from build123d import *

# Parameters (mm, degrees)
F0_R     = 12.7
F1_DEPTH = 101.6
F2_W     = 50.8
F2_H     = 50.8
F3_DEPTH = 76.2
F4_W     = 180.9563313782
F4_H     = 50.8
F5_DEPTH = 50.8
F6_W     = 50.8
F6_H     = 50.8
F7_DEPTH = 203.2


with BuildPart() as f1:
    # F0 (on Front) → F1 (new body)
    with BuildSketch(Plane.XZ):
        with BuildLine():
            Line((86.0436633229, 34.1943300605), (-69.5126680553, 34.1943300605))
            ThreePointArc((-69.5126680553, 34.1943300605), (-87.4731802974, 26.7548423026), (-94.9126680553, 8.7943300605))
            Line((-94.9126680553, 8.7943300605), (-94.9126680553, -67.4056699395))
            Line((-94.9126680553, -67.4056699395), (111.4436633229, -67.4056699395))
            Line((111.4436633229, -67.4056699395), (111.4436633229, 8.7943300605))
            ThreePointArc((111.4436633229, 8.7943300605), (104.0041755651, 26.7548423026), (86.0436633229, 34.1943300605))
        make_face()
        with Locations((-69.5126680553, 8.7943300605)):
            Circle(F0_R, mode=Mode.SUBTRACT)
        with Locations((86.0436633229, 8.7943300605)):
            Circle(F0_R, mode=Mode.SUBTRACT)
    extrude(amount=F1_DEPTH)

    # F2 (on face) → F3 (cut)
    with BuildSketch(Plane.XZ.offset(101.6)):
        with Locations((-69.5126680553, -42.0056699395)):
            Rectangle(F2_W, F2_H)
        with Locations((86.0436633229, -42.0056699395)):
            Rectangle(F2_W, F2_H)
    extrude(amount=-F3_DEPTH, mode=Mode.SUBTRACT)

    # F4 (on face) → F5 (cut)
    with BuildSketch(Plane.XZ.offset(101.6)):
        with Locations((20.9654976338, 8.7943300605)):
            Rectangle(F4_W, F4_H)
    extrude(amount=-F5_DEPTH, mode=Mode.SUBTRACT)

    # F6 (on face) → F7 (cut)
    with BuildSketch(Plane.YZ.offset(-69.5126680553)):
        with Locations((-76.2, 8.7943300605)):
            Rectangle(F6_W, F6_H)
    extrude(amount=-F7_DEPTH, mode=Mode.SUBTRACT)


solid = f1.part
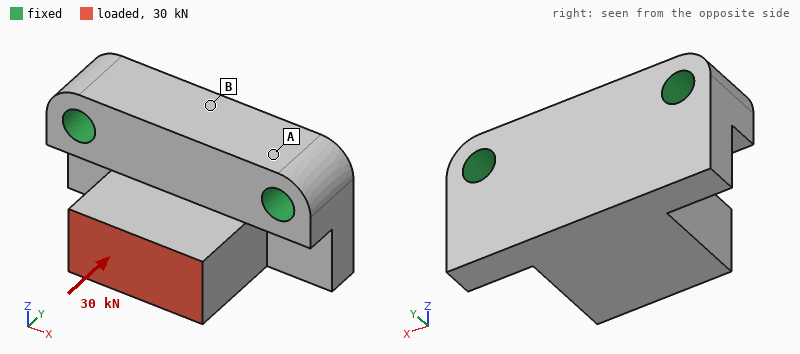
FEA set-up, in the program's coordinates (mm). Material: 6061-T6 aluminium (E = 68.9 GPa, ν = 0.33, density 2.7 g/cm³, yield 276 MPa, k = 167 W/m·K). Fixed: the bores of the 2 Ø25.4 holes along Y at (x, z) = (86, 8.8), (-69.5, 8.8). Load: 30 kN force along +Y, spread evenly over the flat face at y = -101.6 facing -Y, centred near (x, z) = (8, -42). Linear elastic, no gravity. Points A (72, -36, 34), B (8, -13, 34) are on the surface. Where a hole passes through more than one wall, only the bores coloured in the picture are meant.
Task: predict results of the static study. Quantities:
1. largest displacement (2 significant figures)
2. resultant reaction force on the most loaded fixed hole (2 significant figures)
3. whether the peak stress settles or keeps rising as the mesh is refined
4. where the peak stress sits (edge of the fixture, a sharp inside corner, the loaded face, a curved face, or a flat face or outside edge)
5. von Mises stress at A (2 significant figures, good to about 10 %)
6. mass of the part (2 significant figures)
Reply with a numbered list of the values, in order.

1. 99 µm
2. 15 kN
3. keeps rising
4. edge of the fixture
5. 14 MPa
6. 3.1 kg
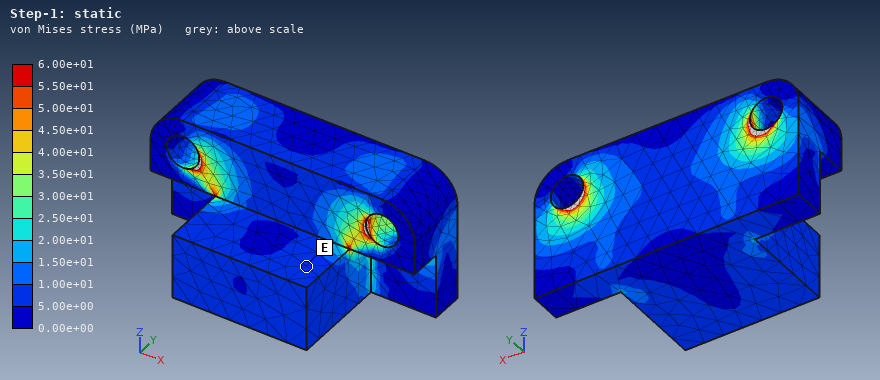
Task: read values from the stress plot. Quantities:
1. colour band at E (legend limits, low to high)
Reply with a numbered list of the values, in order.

1. 5.00e+00 to 1.00e+01 MPa
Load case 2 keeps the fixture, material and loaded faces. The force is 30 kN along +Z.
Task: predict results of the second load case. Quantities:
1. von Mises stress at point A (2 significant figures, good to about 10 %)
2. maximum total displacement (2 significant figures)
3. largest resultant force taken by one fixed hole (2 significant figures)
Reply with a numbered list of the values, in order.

1. 31 MPa
2. 0.23 mm
3. 16 kN
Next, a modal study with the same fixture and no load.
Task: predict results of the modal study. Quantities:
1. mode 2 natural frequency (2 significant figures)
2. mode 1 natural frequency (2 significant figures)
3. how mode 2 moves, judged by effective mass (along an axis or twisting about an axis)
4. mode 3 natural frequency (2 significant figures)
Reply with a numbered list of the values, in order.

1. 4700 Hz
2. 2400 Hz
3. along X
4. 5400 Hz
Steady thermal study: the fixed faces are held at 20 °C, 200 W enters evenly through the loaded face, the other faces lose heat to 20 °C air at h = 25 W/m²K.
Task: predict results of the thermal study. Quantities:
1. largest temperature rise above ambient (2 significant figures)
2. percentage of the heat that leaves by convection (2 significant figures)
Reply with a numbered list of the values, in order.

1. 24 K
2. 7.3 %
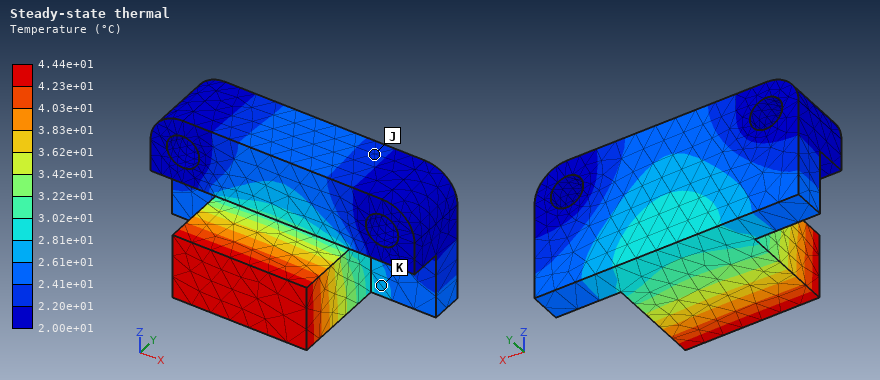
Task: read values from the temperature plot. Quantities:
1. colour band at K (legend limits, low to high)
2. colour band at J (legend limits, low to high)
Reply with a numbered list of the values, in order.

1. 2.61e+01 to 2.81e+01 °C
2. 2.20e+01 to 2.41e+01 °C
